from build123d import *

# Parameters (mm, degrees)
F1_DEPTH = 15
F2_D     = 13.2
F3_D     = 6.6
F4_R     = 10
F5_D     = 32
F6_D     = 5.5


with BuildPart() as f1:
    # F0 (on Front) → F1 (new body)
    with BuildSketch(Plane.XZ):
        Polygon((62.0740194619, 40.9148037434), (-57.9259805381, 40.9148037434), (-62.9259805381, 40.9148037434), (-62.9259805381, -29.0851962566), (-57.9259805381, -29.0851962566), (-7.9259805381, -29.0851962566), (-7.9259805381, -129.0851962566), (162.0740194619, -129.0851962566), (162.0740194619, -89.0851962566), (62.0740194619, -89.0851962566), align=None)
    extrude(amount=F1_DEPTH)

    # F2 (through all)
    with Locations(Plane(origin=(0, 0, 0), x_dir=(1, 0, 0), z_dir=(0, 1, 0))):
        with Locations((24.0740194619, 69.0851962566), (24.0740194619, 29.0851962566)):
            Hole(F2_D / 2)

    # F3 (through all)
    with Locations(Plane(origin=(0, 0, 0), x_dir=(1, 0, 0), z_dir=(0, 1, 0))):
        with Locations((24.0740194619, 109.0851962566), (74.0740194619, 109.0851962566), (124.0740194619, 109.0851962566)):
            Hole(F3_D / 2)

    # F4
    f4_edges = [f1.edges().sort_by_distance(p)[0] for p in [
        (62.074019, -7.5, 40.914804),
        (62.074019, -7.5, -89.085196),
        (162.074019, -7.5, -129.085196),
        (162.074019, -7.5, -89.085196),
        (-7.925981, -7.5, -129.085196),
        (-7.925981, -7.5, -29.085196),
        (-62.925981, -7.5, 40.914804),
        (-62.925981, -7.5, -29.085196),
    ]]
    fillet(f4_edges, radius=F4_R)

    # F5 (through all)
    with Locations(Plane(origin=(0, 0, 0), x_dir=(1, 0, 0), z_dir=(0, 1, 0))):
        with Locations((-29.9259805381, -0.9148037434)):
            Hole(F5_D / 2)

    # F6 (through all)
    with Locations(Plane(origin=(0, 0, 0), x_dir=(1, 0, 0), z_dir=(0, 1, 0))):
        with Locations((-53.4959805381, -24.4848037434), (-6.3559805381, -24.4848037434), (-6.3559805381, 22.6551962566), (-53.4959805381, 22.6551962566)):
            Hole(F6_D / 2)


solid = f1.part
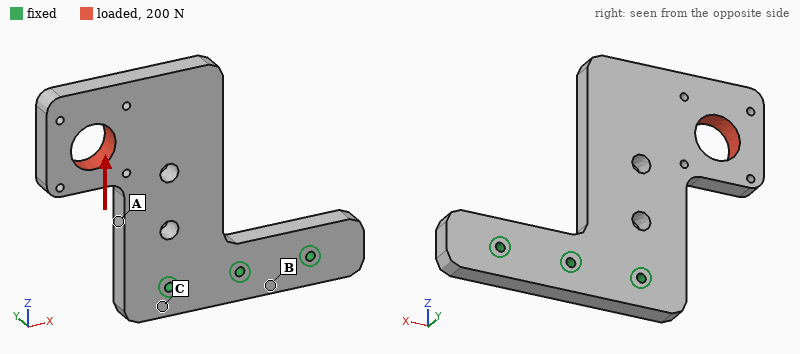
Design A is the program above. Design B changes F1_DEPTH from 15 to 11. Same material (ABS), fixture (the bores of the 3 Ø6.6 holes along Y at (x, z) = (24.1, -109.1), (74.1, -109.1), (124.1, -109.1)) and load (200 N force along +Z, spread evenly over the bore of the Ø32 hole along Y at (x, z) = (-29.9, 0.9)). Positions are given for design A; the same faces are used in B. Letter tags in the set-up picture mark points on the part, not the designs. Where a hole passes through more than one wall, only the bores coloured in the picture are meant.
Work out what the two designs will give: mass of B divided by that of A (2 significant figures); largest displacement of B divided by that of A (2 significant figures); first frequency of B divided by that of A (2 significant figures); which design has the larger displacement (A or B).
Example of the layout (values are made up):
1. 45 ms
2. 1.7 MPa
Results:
1. 0.73
2. 1.4
3. 0.75
4. B
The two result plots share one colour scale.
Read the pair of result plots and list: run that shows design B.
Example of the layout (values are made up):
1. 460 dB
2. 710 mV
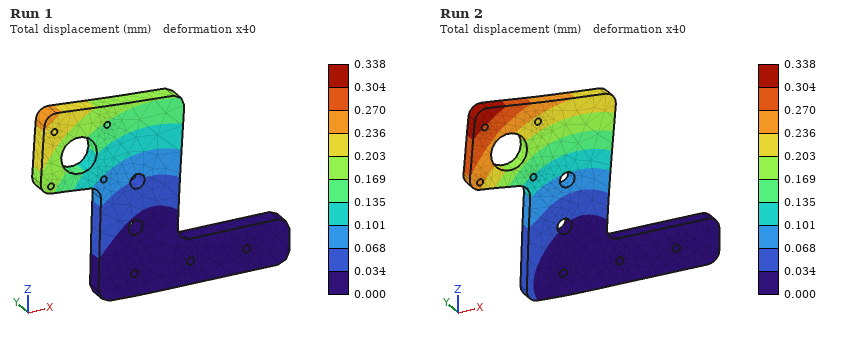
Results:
1. Run 2
